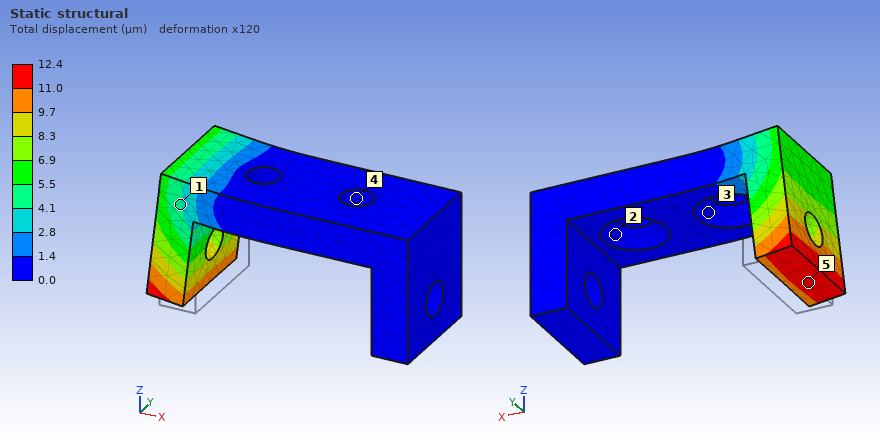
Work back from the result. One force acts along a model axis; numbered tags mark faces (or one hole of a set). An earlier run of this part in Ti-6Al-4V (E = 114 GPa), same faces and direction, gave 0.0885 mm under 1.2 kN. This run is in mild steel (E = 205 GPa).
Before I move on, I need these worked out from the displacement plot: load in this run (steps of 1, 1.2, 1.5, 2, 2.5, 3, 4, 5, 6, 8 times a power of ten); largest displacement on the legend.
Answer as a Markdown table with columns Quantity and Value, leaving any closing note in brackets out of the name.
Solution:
| Quantity | Value |
|---|---|
| load in this run | 300 N |
| largest displacement on the legend | 12.4 µm |
